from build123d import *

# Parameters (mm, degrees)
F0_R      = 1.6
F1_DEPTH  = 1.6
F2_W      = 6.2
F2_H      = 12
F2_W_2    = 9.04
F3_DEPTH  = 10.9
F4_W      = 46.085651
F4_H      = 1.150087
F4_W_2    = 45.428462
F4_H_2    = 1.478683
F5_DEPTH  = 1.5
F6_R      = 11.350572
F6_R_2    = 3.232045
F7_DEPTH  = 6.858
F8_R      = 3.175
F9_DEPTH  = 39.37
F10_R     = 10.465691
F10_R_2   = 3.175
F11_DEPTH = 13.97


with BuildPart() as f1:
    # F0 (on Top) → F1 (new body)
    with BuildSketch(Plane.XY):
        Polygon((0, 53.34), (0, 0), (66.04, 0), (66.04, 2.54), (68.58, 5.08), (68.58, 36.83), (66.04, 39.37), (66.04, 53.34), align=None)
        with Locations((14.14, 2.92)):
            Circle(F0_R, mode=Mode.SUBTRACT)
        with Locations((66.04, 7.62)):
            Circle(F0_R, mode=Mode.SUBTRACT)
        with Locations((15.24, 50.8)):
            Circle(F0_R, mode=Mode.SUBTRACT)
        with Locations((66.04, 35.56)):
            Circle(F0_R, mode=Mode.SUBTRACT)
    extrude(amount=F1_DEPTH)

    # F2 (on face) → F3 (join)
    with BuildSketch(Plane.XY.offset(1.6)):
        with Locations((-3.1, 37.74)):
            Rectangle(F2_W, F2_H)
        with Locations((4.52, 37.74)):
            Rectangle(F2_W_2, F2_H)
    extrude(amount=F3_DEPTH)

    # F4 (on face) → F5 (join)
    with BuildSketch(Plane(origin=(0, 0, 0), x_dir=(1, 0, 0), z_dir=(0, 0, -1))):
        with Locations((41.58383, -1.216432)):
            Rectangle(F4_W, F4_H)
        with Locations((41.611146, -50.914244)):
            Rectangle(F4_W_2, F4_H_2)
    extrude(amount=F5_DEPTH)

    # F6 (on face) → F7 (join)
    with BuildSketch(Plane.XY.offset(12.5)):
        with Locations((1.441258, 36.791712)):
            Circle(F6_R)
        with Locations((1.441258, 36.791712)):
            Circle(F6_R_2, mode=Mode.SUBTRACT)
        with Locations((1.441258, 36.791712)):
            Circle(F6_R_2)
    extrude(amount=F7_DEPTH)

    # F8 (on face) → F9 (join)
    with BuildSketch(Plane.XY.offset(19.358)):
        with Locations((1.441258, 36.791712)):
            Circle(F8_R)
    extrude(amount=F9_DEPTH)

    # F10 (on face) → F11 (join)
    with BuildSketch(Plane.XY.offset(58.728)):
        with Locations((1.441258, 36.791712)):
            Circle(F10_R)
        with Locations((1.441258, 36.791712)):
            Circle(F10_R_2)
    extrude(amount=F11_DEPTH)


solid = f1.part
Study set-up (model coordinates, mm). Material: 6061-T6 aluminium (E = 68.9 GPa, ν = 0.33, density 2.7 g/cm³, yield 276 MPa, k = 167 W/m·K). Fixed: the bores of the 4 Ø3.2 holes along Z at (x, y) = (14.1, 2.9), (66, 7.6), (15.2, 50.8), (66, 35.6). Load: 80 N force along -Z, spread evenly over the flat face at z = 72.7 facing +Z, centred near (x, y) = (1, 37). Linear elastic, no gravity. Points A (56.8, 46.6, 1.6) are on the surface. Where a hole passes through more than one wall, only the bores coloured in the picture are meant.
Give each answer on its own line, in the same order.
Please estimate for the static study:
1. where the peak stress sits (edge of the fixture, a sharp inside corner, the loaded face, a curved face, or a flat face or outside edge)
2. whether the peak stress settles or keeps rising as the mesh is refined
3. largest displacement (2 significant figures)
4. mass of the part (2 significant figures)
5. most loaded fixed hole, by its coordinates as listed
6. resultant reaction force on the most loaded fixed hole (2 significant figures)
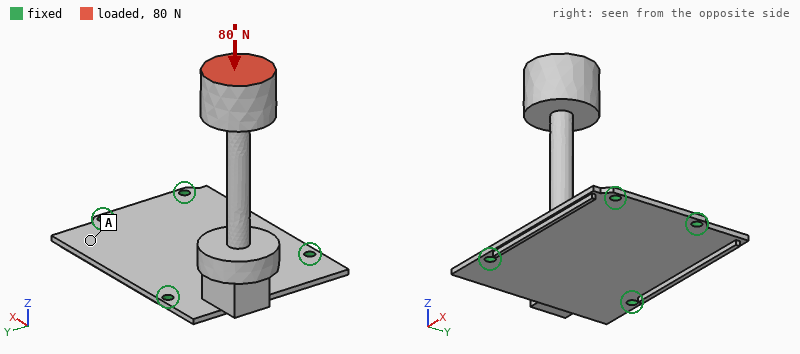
edge of the fixture
keeps rising
0.77 mm
45 g
(15.2, 50.8)
63 N
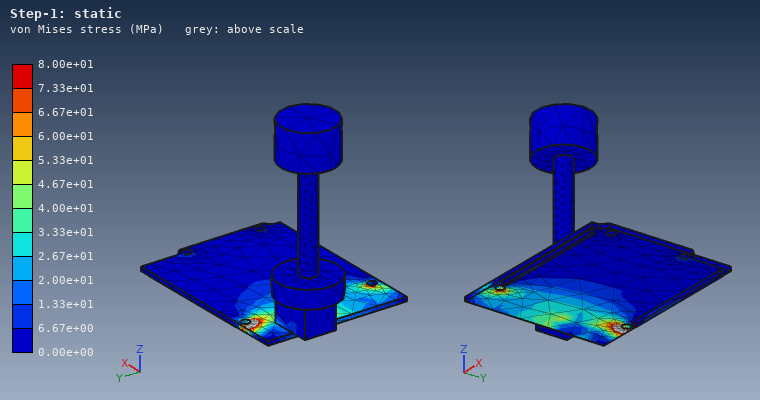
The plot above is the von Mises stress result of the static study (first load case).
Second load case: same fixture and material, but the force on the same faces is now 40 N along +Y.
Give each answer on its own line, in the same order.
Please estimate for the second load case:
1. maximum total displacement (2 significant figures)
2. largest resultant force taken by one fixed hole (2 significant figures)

1.3 mm
76 N
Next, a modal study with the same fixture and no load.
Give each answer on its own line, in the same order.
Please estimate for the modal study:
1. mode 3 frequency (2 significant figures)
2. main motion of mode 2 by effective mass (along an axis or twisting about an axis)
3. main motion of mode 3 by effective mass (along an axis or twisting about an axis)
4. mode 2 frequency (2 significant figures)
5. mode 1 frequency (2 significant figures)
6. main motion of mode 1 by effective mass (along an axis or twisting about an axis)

1200 Hz
along Y
along Z
270 Hz
170 Hz
along X
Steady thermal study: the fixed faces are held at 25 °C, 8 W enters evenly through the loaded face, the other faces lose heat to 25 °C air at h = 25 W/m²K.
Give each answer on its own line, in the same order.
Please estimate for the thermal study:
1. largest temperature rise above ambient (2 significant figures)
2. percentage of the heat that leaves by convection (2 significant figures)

60 K
43 %
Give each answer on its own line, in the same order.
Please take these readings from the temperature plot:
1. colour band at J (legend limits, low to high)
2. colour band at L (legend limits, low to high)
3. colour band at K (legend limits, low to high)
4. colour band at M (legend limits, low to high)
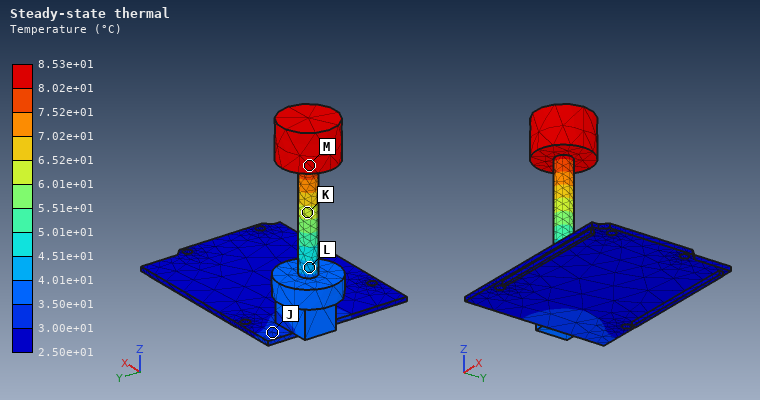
3.00e+01 to 3.50e+01 °C
4.01e+01 to 4.51e+01 °C
6.01e+01 to 6.52e+01 °C
8.02e+01 to 8.53e+01 °C
